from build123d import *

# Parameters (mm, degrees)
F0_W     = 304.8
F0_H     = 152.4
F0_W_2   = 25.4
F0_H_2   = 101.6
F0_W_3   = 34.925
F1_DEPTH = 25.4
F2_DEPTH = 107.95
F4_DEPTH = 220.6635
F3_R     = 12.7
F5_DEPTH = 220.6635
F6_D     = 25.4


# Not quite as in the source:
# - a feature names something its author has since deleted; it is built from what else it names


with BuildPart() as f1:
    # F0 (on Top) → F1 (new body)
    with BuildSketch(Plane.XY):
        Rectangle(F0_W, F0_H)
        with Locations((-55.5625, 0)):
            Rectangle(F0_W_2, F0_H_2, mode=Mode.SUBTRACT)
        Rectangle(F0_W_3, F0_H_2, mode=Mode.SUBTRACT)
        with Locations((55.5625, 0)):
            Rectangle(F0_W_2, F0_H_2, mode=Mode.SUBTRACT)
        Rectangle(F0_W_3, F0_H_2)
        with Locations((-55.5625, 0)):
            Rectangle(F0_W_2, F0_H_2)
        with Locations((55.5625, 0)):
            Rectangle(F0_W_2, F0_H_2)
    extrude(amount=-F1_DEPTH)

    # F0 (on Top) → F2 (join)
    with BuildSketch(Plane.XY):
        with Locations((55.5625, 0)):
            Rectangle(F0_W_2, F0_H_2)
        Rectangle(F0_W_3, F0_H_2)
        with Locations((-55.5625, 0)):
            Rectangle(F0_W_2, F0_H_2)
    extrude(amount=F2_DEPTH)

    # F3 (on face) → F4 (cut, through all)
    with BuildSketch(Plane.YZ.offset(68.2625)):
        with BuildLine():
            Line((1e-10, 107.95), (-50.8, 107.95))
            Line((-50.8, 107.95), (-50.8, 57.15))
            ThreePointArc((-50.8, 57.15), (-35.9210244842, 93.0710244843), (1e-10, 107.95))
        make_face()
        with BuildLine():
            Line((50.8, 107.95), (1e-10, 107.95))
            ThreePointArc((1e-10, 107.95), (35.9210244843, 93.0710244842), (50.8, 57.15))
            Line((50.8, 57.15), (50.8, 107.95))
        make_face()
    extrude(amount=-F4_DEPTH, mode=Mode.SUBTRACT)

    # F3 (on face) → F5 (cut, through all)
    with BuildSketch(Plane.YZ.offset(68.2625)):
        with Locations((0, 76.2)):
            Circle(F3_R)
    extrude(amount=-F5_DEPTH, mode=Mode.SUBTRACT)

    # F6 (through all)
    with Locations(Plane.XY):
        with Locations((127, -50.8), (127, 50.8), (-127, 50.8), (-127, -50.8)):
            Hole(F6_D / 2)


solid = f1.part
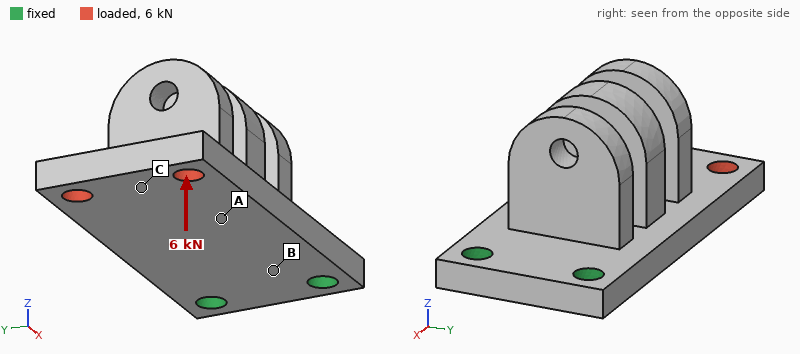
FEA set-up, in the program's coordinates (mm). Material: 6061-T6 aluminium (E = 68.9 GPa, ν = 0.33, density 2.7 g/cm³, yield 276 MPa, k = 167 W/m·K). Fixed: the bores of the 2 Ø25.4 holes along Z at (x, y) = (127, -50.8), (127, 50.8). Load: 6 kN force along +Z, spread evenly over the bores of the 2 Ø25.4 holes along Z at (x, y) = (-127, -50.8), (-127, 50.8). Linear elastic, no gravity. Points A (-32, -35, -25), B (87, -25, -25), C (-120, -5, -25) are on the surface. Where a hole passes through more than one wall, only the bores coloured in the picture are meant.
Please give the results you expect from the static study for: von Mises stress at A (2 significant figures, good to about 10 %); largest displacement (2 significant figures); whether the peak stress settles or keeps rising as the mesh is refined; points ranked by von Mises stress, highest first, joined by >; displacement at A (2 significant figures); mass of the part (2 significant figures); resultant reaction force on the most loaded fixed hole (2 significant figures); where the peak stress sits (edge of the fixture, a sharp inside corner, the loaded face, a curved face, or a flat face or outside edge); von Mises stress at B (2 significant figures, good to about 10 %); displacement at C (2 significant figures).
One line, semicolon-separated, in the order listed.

33 MPa; 2.3 mm; keeps rising; B > A > C; 0.93 mm; 5.2 kg; 3.0 kN; edge of the fixture; 69 MPa; 1.9 mm
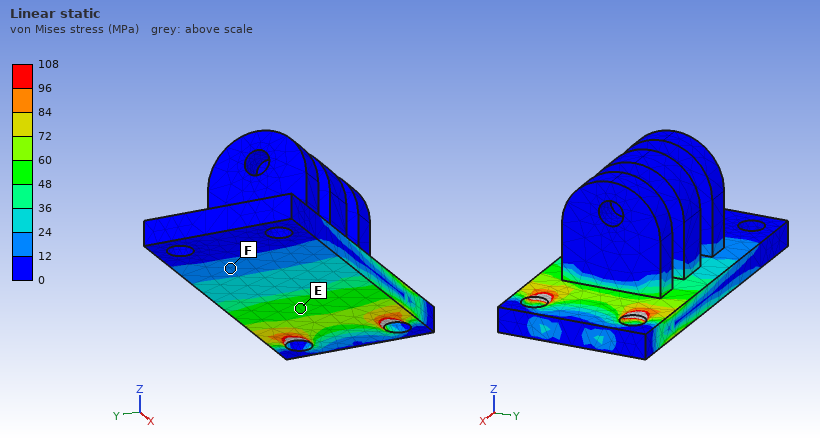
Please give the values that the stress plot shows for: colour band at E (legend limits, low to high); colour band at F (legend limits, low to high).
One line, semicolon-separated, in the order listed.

48 to 60 MPa; 12 to 24 MPa
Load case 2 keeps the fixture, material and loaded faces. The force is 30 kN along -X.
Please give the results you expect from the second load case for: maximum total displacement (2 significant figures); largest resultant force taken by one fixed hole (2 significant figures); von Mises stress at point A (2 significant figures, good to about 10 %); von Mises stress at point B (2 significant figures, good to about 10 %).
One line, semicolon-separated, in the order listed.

46 µm; 15 kN; 7.6 MPa; 7.3 MPa
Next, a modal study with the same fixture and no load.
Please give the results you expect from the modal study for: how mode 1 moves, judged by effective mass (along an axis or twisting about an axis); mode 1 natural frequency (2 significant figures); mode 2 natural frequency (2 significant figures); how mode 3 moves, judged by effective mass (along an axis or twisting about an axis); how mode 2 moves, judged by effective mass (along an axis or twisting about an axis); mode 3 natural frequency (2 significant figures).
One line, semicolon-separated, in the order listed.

along Z; 230 Hz; 750 Hz; along Z; along Y; 1100 Hz
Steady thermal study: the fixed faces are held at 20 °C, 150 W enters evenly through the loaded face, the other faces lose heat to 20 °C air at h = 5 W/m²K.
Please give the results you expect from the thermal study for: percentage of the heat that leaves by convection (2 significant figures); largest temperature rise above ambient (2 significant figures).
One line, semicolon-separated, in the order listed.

15 %; 56 K
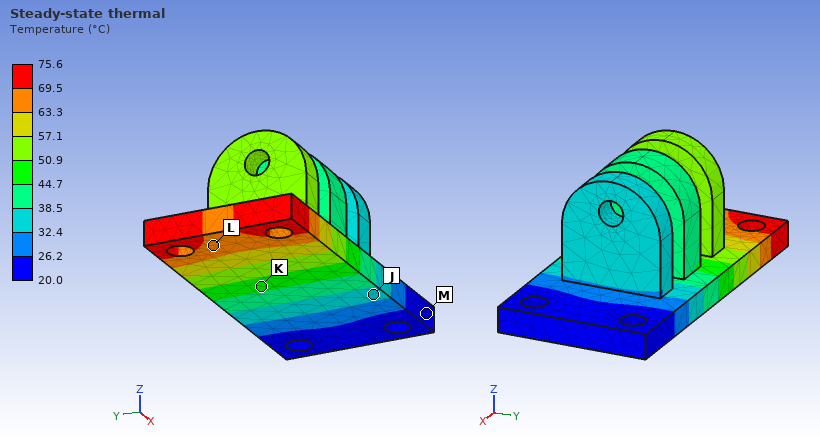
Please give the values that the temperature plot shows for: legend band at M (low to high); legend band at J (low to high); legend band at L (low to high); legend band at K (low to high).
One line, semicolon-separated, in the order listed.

20.0 to 26.2 °C; 32.4 to 38.5 °C; 63.3 to 69.5 °C; 44.7 to 50.9 °C
